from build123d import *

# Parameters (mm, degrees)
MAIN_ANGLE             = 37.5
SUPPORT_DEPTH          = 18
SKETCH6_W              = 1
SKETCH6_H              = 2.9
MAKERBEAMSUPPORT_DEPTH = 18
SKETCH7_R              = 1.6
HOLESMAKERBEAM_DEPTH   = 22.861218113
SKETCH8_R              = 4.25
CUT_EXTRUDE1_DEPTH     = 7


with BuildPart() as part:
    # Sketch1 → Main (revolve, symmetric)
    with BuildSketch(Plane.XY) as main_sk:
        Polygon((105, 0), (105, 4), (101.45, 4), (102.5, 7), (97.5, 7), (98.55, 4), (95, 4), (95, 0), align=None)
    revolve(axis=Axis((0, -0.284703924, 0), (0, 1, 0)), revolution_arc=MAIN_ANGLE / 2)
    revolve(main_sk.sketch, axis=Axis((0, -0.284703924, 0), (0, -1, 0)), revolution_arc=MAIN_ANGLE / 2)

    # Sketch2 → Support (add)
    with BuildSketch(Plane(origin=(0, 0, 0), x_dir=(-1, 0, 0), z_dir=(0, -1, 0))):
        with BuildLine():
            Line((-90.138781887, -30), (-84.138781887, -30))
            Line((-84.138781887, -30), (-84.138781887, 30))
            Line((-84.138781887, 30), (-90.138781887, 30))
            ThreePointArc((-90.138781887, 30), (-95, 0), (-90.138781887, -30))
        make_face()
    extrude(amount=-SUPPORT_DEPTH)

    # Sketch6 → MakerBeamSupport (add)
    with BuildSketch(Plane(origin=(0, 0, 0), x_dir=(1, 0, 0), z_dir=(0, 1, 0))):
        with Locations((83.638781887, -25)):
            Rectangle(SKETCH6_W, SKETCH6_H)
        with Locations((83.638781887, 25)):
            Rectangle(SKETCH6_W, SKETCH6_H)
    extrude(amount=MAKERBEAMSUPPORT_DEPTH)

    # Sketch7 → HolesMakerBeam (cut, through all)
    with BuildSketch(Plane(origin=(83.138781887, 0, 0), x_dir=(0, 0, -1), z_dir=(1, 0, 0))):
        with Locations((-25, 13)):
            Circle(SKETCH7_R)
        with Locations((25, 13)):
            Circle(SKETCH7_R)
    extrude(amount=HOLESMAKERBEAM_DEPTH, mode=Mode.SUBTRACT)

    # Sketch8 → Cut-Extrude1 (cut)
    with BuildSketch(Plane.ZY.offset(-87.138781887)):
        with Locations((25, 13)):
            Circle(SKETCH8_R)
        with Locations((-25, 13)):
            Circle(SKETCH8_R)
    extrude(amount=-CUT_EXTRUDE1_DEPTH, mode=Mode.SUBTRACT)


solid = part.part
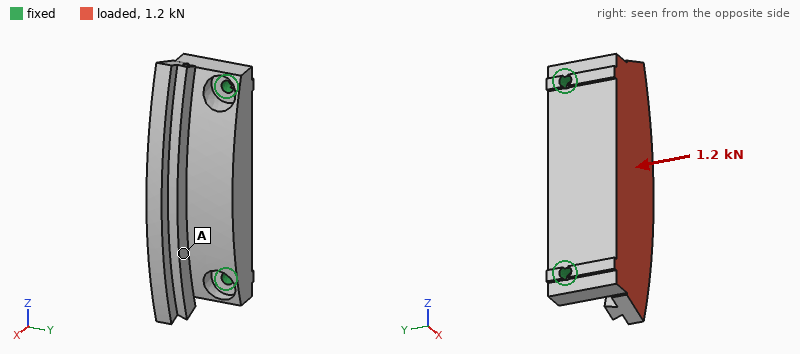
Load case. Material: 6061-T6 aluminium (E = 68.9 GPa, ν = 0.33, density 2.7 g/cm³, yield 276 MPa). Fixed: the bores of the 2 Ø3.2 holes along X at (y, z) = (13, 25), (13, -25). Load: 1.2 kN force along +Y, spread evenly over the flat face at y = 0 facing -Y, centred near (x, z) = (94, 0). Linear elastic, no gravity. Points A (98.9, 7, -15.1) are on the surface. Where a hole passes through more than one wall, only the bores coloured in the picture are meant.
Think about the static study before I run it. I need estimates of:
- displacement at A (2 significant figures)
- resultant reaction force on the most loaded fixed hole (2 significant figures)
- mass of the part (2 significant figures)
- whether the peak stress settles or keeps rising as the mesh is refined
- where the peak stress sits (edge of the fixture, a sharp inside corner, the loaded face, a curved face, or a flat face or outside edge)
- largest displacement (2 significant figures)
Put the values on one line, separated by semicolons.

52 µm; 650 N; 35 g; keeps rising; edge of the fixture; 87 µm
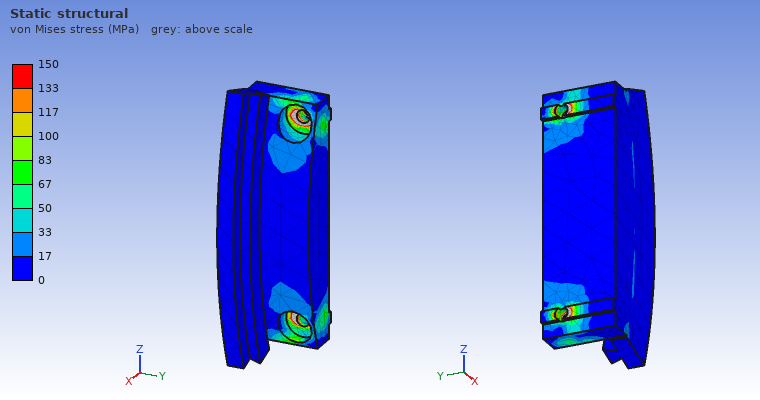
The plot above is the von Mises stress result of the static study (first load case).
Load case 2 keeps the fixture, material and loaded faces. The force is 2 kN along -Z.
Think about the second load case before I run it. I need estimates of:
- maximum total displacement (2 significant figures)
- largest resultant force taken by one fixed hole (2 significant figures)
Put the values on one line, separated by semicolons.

11 µm; 1.2 kN
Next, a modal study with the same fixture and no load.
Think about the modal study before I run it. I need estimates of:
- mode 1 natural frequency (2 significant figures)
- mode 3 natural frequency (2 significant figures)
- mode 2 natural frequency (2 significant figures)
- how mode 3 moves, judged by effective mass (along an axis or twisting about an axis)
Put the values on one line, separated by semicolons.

4400 Hz; 12 kHz; 11 kHz; along X
